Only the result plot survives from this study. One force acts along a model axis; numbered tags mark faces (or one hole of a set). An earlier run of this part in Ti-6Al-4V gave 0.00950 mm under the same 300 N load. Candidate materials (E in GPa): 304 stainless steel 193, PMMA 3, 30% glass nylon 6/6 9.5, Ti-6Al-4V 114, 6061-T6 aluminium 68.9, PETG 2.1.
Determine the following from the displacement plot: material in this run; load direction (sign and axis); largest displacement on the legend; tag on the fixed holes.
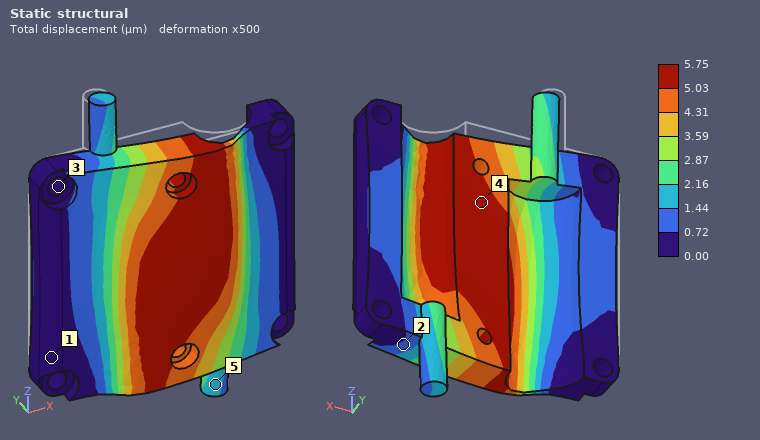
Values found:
304 stainless steel
-Y
5.75 µm
3
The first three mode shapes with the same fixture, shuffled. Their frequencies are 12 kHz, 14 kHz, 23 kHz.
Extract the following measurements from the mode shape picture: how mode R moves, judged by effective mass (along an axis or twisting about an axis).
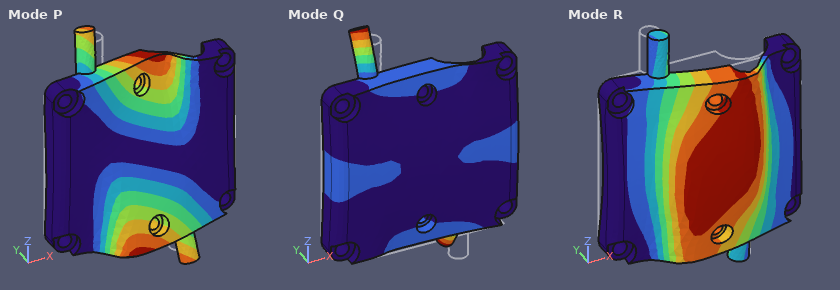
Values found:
along Y
